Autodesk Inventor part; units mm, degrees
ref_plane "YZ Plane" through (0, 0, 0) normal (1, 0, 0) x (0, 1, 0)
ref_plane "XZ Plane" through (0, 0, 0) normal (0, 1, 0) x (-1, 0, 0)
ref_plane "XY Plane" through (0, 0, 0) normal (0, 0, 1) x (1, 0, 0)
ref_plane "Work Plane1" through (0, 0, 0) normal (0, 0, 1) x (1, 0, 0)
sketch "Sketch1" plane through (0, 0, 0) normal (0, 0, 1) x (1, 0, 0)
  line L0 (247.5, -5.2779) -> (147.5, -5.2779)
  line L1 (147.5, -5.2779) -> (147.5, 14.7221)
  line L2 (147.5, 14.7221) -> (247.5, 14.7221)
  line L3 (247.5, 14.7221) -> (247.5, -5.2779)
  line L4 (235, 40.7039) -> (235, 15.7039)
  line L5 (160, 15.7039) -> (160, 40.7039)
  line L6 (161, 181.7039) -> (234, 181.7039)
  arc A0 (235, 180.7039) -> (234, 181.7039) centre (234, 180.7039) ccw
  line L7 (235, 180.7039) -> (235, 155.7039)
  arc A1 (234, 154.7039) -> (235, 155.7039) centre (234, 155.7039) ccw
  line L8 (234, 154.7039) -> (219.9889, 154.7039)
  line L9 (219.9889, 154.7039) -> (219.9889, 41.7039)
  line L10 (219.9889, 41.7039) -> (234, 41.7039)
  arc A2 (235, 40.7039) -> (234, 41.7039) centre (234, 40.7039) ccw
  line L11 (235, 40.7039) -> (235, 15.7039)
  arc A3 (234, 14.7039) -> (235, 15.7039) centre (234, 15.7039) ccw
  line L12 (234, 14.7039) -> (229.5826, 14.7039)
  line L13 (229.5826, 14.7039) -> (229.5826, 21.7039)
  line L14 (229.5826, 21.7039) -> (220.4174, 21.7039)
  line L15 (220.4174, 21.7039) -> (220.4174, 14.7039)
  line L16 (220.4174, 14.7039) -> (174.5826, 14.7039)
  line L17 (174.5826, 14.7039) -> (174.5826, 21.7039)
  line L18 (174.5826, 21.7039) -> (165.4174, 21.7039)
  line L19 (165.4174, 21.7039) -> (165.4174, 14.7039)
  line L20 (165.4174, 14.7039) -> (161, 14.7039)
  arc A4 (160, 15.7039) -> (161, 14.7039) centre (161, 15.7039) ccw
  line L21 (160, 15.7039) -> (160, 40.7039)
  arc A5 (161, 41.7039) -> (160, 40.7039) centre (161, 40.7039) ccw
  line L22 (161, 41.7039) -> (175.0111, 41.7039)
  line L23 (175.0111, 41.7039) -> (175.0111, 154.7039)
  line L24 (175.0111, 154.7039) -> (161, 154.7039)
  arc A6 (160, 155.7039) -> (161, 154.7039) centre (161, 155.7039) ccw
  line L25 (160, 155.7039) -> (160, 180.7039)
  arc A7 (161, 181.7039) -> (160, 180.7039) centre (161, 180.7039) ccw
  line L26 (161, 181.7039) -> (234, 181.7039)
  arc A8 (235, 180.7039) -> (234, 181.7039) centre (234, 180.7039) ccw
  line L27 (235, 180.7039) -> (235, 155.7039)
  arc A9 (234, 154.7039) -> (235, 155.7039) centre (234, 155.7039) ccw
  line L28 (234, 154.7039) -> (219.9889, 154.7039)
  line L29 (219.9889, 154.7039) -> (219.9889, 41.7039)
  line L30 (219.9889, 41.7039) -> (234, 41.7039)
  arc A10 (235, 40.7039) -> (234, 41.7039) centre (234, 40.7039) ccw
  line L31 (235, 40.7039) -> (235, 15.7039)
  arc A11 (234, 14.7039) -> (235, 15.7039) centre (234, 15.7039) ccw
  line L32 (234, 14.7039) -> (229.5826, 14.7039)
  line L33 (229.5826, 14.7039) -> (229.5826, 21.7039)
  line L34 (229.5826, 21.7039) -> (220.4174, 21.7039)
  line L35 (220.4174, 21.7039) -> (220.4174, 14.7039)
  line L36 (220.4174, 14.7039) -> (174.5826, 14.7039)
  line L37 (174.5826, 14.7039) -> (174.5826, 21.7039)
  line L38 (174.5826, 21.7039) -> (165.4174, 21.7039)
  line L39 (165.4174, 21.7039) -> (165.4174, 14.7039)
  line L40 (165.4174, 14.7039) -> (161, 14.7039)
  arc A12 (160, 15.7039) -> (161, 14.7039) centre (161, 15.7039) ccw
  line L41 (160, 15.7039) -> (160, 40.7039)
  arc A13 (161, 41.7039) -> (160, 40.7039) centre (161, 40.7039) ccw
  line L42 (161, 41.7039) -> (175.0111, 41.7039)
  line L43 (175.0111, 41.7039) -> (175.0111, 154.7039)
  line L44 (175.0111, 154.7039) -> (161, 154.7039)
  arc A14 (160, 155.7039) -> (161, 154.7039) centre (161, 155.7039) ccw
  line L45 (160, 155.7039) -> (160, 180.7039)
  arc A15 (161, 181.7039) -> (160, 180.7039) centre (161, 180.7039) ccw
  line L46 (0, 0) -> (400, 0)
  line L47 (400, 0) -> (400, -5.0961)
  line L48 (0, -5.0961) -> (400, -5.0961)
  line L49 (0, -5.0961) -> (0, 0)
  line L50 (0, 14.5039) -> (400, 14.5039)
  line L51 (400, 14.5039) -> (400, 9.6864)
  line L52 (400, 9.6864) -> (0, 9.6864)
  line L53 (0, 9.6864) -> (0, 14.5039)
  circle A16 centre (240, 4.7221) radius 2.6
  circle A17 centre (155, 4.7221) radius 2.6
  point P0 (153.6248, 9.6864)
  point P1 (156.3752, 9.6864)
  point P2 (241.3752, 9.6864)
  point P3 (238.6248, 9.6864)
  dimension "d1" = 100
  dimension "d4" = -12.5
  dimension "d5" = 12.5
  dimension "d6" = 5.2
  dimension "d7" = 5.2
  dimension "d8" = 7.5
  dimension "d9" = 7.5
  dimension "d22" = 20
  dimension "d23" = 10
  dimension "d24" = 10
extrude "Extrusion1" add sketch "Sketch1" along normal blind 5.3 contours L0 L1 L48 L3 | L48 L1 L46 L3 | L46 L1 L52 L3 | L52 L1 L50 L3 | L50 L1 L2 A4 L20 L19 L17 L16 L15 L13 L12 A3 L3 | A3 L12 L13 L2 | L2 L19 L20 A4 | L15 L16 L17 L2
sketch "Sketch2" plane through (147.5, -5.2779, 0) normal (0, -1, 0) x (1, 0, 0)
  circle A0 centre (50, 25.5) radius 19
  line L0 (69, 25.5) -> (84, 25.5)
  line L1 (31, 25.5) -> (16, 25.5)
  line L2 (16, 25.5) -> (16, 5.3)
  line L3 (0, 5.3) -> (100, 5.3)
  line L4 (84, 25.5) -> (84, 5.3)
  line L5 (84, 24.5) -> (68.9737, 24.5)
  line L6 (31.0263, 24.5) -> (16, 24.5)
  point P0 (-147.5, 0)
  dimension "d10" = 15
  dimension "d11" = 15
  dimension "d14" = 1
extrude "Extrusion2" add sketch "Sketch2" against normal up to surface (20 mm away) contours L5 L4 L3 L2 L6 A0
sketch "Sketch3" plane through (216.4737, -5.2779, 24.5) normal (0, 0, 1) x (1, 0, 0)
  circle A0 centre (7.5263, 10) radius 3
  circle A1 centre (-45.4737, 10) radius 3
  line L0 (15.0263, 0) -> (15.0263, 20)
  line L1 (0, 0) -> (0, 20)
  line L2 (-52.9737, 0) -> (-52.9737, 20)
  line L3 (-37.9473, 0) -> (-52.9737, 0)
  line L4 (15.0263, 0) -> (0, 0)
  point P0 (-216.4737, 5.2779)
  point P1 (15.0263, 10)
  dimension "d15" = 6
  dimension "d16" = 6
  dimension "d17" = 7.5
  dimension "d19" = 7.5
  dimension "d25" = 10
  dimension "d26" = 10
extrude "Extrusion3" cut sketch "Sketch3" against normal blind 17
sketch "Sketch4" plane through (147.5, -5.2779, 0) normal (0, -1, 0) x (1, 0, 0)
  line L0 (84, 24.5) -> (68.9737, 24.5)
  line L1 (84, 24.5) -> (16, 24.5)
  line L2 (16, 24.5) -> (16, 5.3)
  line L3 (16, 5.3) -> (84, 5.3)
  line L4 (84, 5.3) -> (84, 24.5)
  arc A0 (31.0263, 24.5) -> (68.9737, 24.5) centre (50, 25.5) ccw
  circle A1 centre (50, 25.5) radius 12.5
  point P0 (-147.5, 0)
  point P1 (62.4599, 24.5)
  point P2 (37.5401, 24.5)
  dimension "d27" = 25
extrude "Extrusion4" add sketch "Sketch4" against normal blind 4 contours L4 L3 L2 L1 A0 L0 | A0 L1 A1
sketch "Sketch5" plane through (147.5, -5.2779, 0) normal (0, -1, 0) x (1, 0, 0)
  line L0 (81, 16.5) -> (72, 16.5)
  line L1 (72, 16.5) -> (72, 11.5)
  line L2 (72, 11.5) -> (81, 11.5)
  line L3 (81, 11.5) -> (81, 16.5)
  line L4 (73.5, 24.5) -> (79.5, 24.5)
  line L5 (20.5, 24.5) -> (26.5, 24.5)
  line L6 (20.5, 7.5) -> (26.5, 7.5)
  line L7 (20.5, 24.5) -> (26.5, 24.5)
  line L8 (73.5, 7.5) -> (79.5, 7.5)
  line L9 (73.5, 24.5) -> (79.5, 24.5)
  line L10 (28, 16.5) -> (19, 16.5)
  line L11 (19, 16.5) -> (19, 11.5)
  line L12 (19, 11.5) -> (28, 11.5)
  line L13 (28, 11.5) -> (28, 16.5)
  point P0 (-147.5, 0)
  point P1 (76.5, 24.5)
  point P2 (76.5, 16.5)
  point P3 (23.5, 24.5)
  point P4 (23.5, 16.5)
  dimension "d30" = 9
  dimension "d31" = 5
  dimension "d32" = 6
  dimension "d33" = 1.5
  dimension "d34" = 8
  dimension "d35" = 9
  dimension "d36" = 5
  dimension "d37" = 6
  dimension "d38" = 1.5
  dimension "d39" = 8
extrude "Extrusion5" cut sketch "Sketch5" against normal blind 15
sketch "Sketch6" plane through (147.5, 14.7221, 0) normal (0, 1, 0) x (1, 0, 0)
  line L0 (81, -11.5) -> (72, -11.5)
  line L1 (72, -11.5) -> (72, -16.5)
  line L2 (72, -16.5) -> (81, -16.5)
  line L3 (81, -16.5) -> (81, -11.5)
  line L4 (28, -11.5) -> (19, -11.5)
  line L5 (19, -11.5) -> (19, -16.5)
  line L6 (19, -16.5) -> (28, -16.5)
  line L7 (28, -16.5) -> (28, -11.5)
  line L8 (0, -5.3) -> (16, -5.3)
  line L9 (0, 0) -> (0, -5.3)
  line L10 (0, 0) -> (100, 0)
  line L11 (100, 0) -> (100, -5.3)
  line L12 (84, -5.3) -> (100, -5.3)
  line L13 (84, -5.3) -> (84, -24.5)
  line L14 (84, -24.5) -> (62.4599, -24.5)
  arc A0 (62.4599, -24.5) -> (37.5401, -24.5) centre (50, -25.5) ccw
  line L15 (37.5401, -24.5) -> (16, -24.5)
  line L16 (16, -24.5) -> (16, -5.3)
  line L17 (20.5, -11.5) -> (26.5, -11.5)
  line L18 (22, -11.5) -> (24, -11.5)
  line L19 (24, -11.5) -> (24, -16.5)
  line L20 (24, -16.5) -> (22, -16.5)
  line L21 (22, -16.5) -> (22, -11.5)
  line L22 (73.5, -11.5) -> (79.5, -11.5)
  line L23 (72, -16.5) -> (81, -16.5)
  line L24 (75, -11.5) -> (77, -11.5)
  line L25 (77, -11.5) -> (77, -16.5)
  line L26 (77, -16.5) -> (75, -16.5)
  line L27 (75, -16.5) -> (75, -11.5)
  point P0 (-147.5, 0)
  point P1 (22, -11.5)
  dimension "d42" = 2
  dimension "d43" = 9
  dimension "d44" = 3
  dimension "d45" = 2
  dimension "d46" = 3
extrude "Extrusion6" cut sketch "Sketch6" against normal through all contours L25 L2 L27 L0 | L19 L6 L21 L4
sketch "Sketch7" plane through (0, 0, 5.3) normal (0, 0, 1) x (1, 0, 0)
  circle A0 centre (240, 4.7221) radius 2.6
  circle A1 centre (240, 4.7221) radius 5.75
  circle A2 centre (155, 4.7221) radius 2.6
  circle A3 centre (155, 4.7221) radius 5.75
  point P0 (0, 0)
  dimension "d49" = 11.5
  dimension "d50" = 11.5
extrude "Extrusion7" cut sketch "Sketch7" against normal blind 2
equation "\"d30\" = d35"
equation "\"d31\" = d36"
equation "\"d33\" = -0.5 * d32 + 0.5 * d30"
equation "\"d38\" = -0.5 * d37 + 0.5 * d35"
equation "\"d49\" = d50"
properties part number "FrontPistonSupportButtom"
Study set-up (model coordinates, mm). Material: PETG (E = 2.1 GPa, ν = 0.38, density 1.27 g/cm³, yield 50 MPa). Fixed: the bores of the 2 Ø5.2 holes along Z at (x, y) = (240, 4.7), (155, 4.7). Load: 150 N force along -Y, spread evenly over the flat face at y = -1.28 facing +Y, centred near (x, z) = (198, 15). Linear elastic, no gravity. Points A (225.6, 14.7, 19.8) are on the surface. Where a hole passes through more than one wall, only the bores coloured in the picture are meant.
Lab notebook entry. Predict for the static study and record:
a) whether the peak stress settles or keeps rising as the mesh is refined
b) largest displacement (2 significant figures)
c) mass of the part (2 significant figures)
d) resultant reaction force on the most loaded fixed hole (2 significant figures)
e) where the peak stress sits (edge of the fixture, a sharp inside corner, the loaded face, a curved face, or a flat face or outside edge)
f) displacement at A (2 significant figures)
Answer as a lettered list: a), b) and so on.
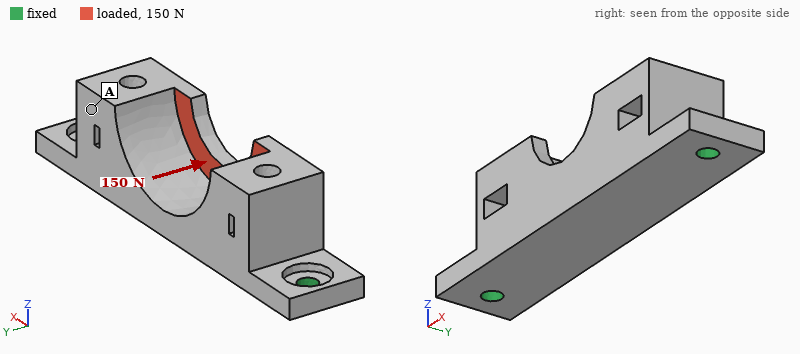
a) keeps rising
b) 0.59 mm
c) 31 g
d) 75 N
e) edge of the fixture
f) 0.43 mm
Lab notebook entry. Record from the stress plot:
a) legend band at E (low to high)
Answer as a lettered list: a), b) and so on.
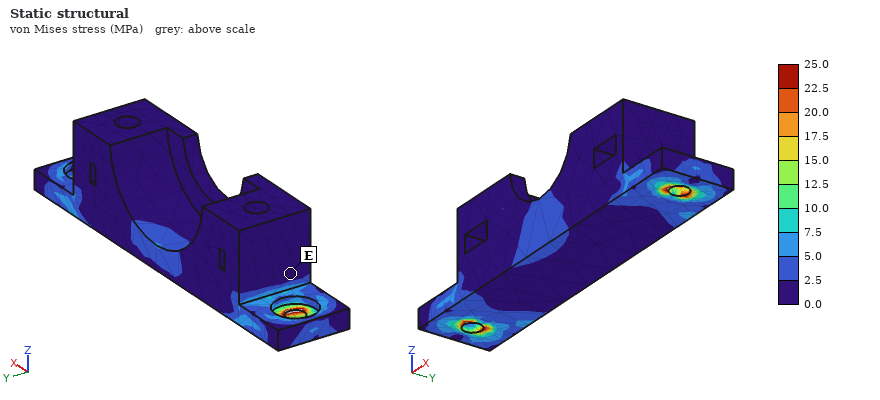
a) 0.0 to 2.5 MPa
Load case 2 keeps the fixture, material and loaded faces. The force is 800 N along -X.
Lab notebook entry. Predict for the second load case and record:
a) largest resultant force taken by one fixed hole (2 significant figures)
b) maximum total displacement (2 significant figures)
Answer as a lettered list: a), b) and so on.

a) 430 N
b) 0.16 mm
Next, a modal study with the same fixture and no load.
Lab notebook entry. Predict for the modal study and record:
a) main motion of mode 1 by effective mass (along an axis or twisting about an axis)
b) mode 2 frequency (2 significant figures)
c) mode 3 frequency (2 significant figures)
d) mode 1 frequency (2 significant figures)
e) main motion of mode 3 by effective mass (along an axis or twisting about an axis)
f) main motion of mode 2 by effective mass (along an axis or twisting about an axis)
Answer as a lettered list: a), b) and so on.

a) along Y
b) 1000 Hz
c) 1600 Hz
d) 750 Hz
e) twisting about Z
f) along Z
